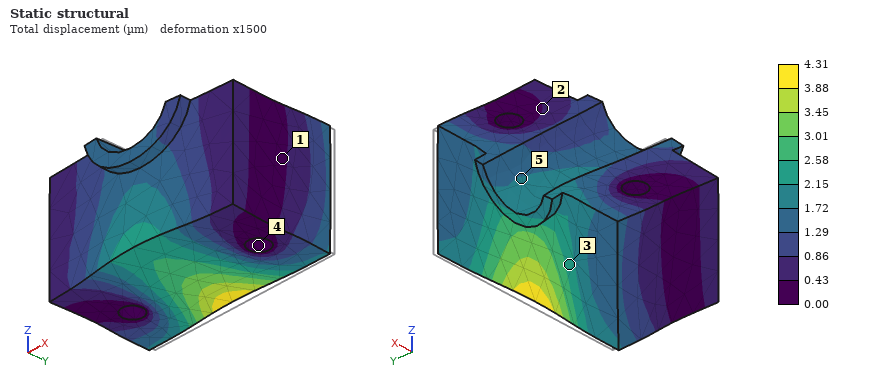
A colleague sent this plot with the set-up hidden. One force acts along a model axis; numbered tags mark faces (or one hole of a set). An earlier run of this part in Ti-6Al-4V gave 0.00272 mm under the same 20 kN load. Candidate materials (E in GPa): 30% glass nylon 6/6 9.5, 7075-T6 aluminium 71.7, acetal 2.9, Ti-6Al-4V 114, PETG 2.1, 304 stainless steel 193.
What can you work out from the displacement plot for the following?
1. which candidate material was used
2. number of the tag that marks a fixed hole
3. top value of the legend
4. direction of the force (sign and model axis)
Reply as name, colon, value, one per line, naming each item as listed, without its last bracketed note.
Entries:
which candidate material was used: 7075-T6 aluminium
number of the tag that marks a fixed hole: 4
top value of the legend: 4.31 µm
direction of the force: -Y
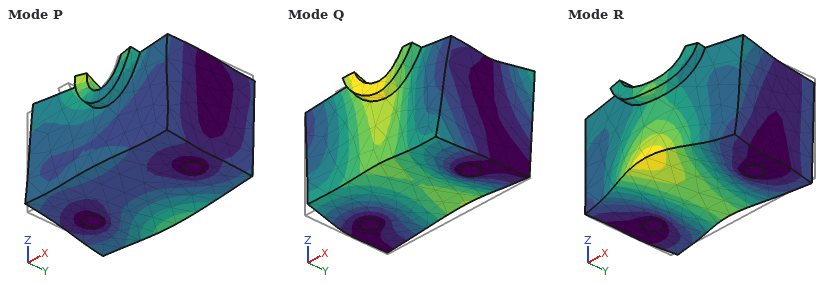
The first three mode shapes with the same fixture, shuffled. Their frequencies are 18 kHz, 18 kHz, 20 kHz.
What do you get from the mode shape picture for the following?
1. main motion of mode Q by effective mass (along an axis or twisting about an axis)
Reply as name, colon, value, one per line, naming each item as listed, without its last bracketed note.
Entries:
main motion of mode Q by effective mass: along Z
